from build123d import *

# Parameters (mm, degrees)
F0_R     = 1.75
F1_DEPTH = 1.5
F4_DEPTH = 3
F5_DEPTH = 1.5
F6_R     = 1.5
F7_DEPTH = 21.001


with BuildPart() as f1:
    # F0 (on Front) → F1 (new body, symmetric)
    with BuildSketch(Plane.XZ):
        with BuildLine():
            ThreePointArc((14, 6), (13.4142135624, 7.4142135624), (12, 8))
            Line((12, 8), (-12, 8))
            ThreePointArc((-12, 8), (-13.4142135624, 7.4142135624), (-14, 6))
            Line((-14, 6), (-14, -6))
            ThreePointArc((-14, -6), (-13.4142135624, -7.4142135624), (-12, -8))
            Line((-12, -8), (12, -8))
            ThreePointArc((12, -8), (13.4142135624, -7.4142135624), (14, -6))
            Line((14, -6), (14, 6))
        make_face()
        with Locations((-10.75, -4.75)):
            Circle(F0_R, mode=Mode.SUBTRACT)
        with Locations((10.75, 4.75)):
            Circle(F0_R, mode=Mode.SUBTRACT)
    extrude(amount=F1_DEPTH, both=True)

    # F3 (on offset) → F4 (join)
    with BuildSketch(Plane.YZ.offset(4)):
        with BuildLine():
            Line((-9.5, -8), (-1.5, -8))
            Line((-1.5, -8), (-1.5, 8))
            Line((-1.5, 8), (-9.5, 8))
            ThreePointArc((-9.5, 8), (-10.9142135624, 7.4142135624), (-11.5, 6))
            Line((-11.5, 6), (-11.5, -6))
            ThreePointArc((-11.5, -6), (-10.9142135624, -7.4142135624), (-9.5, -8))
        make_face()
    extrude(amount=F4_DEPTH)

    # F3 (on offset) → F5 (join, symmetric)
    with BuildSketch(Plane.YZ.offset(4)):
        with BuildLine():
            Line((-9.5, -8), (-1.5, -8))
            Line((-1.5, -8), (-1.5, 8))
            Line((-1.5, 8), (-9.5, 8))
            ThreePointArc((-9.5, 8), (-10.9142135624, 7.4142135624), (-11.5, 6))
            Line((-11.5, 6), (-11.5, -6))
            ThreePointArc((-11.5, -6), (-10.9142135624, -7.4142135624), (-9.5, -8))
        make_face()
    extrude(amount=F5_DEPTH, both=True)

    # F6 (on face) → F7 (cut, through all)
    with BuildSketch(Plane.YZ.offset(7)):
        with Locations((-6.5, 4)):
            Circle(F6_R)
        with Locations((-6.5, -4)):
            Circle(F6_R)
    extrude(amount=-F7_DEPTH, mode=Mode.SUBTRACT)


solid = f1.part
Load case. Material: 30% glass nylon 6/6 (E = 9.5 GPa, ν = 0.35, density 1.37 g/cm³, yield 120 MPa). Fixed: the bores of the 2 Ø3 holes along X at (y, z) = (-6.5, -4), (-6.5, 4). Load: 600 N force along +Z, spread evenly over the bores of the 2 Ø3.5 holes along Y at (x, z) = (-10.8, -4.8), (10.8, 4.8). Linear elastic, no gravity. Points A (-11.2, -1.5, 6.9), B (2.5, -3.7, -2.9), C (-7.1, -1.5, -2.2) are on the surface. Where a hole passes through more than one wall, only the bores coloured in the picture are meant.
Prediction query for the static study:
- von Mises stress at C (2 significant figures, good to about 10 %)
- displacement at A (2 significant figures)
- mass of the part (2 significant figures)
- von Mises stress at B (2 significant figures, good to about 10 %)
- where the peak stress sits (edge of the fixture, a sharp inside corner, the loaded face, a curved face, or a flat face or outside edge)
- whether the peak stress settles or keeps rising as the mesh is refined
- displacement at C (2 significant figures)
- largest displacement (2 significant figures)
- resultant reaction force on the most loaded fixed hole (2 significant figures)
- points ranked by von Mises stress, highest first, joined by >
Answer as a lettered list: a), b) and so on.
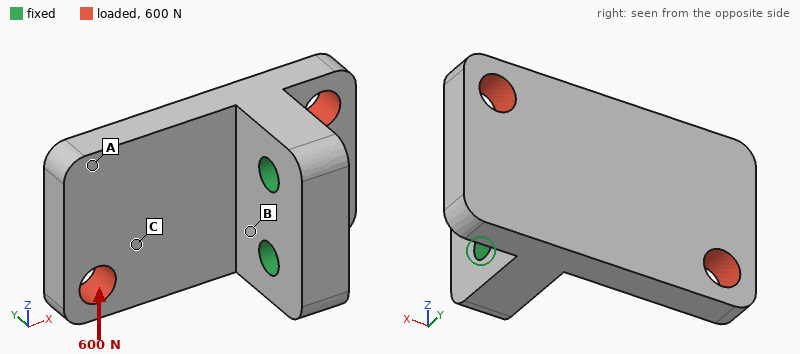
a) 19 MPa
b) 0.17 mm
c) 2.6 g
d) 41 MPa
e) edge of the fixture
f) keeps rising
g) 0.12 mm
h) 0.21 mm
i) 510 N
j) B > C > A
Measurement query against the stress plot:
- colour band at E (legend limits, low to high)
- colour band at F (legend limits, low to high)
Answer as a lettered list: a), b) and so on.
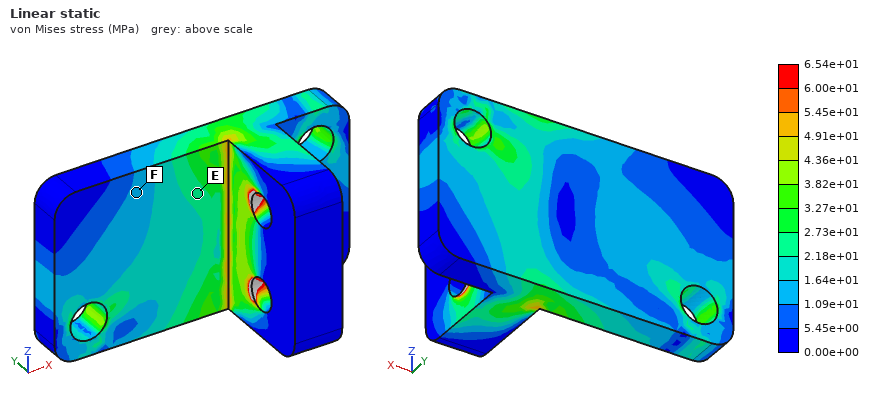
a) 2.18e+01 to 2.73e+01 MPa
b) 1.09e+01 to 1.64e+01 MPa
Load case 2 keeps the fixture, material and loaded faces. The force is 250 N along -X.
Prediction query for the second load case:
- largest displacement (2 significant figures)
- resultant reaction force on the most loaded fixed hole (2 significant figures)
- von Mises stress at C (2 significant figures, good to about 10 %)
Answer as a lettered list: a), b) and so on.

a) 89 µm
b) 130 N
c) 4.7 MPa
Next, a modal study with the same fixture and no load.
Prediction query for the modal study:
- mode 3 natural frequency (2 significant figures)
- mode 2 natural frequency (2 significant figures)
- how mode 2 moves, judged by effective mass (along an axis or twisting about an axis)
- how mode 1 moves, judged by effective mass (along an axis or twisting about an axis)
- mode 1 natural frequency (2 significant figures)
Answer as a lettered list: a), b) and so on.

a) 10000 Hz
b) 7500 Hz
c) along Z
d) along Y
e) 3600 Hz
